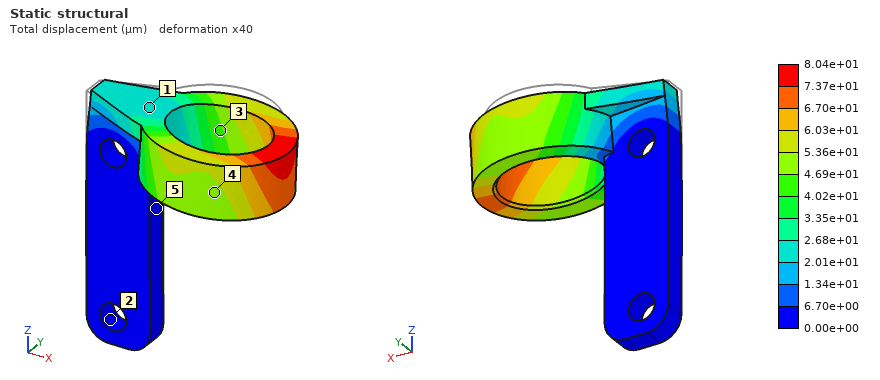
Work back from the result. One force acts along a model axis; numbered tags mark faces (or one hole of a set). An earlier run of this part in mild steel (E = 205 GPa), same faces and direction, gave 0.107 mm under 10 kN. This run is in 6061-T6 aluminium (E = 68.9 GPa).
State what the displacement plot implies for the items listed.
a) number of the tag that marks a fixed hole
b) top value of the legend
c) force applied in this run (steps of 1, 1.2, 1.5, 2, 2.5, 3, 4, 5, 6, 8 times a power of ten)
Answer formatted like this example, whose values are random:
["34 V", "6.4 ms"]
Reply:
["2", "8.04e+01 µm", "2.5 kN"]
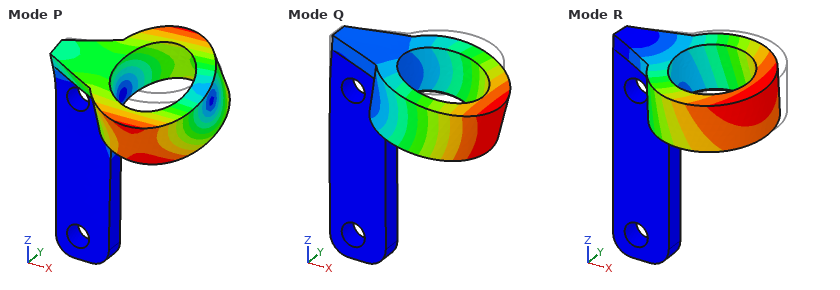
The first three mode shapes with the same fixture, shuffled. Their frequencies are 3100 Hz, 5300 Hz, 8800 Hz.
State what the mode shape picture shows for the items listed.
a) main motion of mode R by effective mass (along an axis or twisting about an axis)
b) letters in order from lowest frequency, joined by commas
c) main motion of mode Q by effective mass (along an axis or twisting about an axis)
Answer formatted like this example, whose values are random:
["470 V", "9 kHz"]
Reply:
["along Y", "R, Q, P", "along Z"]
